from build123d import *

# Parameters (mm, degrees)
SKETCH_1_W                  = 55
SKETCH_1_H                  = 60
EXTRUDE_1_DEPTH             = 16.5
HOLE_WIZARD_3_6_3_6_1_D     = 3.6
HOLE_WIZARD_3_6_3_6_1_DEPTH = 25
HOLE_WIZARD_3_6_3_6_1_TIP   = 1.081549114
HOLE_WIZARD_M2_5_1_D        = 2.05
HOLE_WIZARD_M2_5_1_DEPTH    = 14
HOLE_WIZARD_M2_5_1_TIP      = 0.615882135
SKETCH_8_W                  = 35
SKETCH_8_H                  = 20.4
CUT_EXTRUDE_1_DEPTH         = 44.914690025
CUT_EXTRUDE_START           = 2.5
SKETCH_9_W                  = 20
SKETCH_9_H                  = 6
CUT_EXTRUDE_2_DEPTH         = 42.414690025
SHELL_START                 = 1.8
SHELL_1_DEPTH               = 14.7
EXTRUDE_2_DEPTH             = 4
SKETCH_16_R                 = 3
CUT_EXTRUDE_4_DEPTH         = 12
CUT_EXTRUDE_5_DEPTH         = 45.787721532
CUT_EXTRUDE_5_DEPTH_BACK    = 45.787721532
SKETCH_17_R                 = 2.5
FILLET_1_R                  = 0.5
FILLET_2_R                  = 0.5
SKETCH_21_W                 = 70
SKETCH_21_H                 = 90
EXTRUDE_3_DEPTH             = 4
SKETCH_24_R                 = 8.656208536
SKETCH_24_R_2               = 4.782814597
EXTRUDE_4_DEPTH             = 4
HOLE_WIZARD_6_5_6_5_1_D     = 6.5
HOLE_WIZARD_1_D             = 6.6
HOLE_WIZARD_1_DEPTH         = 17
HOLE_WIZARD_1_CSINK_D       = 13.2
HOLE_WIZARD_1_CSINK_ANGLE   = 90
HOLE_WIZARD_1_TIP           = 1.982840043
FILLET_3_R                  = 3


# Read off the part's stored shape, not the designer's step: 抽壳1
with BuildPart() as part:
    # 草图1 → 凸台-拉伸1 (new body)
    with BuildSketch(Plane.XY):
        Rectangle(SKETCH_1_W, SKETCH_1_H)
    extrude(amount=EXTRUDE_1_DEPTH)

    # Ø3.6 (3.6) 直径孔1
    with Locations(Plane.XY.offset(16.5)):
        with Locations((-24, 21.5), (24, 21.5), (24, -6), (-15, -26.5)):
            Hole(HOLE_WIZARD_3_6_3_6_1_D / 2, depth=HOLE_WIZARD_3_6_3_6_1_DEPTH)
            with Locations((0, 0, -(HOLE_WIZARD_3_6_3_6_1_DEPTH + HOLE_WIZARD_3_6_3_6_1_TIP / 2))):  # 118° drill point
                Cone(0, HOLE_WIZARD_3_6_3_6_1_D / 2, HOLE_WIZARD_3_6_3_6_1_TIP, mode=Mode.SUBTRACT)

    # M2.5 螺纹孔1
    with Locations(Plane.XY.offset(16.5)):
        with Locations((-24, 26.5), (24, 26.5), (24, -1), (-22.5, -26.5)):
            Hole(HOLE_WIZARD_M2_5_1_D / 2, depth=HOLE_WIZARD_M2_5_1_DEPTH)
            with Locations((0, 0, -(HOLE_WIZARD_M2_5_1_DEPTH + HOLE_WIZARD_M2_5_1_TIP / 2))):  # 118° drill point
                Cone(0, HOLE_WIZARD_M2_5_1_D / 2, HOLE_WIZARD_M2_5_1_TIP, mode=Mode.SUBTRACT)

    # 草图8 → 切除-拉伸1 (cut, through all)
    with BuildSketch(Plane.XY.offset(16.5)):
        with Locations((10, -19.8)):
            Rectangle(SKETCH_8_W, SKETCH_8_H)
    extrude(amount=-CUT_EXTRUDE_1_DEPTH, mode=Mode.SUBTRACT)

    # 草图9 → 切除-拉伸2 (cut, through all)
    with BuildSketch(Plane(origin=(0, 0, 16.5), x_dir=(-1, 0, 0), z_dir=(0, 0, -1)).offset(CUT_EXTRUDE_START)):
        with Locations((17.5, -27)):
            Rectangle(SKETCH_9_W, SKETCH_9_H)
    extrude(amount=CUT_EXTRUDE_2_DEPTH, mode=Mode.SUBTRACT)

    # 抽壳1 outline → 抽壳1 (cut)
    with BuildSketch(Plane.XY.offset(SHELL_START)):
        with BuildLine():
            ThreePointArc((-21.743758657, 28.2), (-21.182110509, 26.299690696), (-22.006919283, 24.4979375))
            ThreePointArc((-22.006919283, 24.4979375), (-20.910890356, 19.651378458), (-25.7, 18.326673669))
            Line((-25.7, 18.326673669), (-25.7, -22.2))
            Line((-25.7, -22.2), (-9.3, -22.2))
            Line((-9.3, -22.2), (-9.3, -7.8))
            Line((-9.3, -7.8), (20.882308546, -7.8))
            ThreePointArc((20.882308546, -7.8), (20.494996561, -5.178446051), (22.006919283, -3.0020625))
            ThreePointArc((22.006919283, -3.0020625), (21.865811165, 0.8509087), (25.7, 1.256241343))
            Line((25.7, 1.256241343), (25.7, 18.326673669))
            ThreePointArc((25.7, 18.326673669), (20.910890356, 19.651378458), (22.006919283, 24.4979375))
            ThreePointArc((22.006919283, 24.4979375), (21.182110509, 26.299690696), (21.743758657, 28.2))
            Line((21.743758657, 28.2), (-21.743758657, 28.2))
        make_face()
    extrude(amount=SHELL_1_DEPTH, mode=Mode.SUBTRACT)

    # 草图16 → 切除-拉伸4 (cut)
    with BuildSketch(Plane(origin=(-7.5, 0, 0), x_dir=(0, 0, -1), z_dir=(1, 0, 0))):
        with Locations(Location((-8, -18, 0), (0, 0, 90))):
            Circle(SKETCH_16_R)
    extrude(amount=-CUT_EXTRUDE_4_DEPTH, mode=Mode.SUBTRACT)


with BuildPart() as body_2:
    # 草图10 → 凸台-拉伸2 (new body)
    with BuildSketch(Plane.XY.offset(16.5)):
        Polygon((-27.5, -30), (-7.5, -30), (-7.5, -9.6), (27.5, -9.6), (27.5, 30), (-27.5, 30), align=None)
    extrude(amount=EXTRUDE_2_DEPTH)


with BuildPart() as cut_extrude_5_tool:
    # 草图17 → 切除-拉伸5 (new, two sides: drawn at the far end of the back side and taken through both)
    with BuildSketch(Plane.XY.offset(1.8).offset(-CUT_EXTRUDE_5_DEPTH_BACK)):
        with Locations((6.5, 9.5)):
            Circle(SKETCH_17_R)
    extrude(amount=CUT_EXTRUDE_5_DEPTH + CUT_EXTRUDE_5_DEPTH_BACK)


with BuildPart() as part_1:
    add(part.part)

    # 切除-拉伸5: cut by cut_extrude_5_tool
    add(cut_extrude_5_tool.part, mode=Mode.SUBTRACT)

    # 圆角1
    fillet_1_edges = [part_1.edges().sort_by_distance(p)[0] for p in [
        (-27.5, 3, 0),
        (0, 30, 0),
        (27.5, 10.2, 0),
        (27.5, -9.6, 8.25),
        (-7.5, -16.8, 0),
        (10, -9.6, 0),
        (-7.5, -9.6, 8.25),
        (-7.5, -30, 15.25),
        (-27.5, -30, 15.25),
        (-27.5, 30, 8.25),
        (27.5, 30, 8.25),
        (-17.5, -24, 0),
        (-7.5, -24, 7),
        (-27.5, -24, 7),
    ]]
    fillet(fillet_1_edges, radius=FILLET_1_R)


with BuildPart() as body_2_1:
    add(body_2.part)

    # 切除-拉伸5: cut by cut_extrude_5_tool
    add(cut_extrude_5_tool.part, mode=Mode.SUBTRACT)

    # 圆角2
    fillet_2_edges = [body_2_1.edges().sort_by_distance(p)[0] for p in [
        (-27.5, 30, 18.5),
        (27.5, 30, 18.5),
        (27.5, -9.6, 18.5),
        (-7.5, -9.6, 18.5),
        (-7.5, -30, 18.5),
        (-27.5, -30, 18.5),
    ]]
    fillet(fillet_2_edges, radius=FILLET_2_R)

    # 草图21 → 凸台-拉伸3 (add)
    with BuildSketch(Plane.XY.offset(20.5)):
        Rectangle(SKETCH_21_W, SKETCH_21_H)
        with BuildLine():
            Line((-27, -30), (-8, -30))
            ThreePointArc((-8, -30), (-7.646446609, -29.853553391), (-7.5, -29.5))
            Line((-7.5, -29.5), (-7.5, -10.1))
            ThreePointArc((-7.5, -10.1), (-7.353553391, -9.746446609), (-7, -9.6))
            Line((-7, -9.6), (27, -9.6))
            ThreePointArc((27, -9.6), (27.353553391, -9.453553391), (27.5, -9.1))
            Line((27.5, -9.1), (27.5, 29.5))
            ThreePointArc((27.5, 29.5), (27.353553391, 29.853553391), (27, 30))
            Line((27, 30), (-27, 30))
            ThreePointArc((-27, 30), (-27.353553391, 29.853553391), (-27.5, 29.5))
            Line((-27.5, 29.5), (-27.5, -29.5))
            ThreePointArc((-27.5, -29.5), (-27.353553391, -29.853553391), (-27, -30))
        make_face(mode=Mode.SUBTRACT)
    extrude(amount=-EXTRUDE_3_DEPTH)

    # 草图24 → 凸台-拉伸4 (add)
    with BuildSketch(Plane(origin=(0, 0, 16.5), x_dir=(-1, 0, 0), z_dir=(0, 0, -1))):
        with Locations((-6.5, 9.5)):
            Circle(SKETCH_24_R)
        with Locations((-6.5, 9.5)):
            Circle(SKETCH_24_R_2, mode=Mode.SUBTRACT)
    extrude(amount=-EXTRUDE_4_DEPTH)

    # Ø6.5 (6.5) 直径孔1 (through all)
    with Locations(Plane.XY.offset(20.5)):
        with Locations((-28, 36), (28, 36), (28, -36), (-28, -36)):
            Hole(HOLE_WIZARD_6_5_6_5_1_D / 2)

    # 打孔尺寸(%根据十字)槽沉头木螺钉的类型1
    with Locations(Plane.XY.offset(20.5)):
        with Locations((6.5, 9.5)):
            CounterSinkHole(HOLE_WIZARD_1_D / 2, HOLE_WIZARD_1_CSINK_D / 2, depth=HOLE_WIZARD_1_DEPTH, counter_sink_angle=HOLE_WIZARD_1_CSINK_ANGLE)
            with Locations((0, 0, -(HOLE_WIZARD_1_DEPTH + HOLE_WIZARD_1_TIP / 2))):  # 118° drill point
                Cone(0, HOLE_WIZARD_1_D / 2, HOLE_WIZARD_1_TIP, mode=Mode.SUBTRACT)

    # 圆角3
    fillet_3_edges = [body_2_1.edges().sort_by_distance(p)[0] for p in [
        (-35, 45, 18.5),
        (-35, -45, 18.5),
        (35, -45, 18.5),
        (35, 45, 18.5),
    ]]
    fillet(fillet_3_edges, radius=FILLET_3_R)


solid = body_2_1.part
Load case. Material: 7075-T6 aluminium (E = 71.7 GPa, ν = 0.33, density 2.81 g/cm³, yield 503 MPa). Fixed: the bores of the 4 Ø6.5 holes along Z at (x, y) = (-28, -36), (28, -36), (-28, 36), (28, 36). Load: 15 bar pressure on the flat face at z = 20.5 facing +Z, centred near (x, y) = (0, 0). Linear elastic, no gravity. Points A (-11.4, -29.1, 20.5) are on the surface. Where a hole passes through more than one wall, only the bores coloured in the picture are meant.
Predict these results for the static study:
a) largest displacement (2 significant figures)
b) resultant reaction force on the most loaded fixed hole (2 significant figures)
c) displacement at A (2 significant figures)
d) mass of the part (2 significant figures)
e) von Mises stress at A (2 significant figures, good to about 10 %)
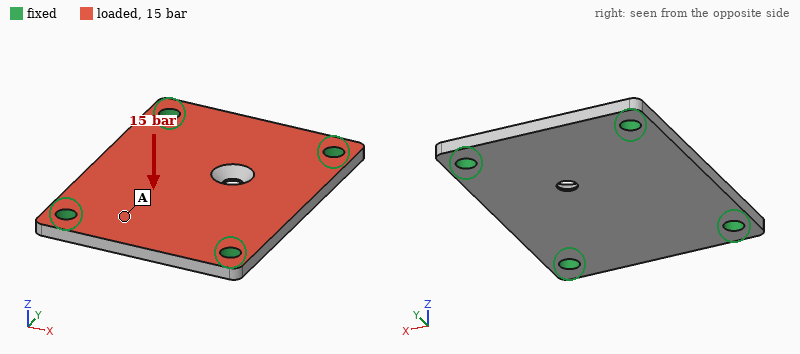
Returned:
0.39 mm
2.3 kN
0.14 mm
68 g
68 MPa
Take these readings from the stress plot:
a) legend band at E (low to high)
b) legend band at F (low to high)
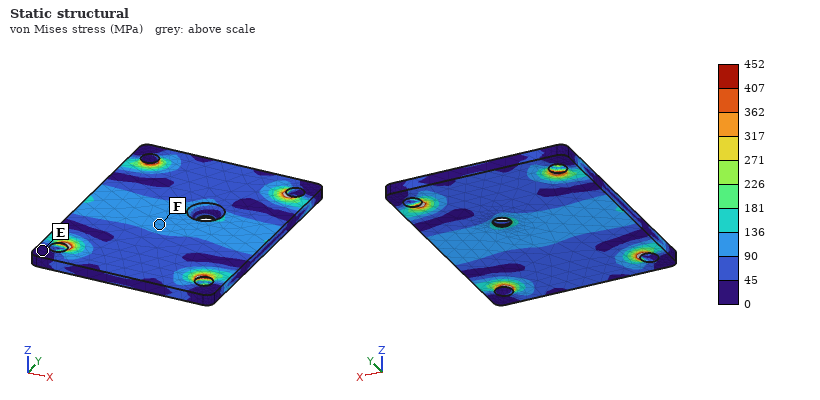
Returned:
0 to 45 MPa
90 to 136 MPa
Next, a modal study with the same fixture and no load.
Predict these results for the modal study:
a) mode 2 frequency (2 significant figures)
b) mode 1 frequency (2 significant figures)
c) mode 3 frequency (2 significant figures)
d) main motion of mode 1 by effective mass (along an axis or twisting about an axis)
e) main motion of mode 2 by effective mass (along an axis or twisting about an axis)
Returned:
5100 Hz
3500 Hz
6700 Hz
along Z
twisting about Y
